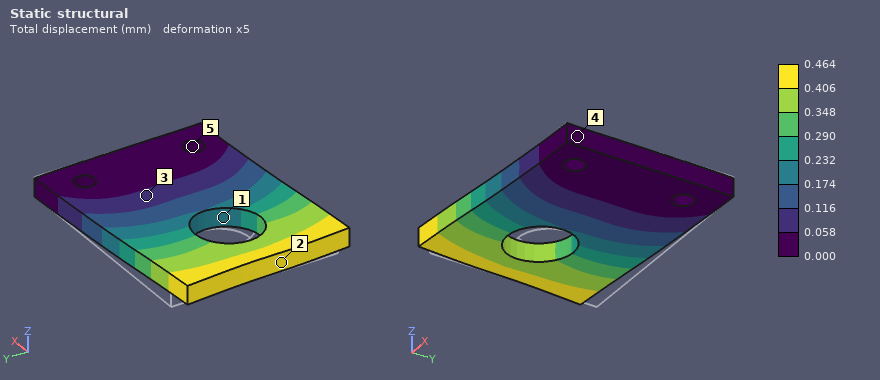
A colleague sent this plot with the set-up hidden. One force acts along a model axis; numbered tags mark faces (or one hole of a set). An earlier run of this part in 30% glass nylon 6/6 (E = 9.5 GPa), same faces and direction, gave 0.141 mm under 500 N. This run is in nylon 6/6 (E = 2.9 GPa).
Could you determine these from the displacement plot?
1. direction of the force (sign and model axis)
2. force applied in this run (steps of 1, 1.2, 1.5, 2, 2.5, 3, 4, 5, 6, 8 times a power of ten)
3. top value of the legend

-Y
500 N
0.464 mm
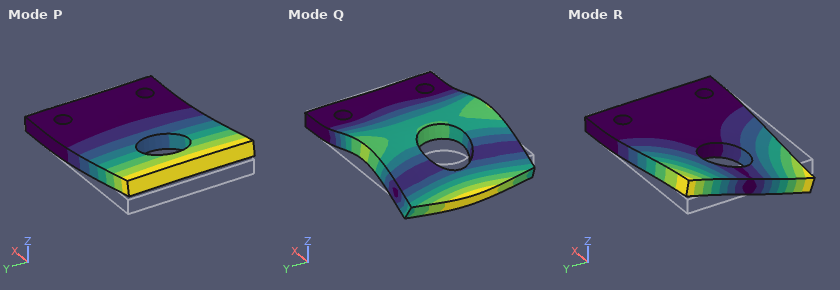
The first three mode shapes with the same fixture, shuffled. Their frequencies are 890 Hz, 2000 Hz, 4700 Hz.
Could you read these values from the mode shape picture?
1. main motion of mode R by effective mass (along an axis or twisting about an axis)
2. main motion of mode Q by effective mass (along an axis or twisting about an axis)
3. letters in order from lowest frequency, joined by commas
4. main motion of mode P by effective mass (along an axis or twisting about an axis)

twisting about X
along Z
P, R, Q
along Z
